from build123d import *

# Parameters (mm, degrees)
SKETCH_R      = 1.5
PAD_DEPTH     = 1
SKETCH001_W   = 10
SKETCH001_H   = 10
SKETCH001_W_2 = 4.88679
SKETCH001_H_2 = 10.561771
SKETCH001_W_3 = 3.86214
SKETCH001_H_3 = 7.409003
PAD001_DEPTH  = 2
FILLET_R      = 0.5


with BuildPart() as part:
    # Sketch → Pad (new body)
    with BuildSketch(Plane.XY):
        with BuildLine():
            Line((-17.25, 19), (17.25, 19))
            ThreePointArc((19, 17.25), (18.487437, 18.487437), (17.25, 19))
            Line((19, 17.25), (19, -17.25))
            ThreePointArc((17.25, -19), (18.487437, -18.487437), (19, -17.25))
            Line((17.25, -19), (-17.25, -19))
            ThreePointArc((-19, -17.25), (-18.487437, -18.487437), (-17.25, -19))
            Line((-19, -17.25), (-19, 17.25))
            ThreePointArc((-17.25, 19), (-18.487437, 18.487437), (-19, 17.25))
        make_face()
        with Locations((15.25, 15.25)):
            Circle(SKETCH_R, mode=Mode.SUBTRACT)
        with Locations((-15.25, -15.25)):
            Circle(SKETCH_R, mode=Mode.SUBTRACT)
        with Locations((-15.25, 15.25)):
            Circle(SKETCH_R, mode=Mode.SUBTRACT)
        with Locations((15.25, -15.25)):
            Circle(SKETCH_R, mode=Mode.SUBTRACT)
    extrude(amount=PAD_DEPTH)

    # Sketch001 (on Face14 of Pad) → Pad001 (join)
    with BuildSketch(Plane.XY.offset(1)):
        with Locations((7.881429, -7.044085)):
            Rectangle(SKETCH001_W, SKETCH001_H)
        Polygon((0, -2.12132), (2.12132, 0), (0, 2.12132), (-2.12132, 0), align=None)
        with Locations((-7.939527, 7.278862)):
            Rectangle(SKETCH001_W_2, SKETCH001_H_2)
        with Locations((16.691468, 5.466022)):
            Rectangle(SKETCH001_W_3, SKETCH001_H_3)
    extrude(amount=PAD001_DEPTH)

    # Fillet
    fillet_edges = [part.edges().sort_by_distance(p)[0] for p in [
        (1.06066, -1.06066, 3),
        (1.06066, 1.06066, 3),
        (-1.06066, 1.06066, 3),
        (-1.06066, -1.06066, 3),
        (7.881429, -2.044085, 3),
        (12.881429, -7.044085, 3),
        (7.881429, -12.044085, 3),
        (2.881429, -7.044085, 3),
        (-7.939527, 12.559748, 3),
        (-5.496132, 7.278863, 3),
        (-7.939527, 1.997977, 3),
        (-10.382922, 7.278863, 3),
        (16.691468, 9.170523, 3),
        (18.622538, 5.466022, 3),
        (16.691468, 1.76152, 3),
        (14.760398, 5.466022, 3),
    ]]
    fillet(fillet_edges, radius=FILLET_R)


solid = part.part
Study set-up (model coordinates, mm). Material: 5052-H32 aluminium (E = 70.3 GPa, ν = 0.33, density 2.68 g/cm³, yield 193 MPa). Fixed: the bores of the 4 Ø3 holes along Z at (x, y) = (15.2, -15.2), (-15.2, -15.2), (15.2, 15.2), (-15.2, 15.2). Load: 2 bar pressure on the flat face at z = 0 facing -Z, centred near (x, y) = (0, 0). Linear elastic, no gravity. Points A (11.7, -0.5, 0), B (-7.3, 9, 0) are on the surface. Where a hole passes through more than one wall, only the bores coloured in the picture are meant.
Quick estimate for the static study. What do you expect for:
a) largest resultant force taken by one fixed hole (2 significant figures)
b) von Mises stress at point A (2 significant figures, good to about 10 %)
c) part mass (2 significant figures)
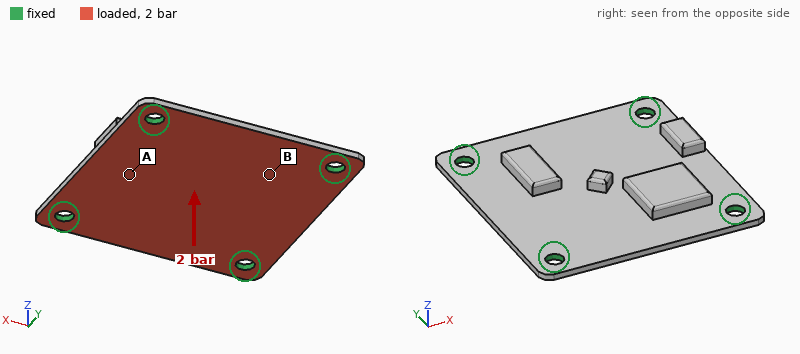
78 N
56 MPa
4.8 g
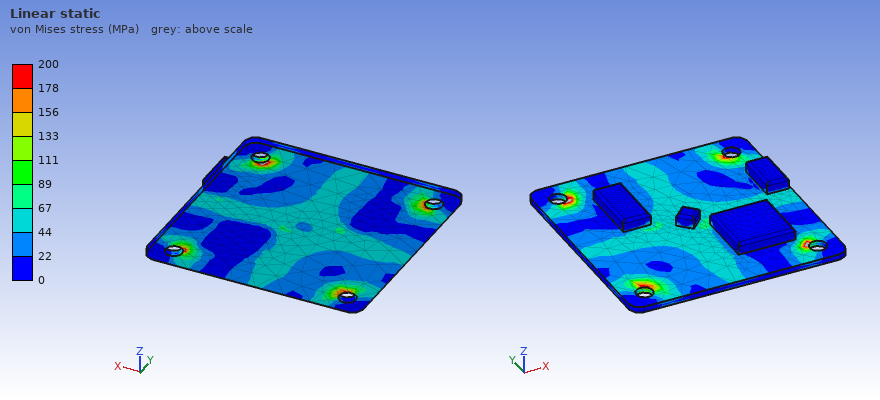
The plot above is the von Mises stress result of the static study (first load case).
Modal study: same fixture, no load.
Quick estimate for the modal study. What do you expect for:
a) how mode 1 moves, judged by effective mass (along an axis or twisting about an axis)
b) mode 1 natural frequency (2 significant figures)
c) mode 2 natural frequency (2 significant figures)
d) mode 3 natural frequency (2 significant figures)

along Z
4000 Hz
6800 Hz
7500 Hz
